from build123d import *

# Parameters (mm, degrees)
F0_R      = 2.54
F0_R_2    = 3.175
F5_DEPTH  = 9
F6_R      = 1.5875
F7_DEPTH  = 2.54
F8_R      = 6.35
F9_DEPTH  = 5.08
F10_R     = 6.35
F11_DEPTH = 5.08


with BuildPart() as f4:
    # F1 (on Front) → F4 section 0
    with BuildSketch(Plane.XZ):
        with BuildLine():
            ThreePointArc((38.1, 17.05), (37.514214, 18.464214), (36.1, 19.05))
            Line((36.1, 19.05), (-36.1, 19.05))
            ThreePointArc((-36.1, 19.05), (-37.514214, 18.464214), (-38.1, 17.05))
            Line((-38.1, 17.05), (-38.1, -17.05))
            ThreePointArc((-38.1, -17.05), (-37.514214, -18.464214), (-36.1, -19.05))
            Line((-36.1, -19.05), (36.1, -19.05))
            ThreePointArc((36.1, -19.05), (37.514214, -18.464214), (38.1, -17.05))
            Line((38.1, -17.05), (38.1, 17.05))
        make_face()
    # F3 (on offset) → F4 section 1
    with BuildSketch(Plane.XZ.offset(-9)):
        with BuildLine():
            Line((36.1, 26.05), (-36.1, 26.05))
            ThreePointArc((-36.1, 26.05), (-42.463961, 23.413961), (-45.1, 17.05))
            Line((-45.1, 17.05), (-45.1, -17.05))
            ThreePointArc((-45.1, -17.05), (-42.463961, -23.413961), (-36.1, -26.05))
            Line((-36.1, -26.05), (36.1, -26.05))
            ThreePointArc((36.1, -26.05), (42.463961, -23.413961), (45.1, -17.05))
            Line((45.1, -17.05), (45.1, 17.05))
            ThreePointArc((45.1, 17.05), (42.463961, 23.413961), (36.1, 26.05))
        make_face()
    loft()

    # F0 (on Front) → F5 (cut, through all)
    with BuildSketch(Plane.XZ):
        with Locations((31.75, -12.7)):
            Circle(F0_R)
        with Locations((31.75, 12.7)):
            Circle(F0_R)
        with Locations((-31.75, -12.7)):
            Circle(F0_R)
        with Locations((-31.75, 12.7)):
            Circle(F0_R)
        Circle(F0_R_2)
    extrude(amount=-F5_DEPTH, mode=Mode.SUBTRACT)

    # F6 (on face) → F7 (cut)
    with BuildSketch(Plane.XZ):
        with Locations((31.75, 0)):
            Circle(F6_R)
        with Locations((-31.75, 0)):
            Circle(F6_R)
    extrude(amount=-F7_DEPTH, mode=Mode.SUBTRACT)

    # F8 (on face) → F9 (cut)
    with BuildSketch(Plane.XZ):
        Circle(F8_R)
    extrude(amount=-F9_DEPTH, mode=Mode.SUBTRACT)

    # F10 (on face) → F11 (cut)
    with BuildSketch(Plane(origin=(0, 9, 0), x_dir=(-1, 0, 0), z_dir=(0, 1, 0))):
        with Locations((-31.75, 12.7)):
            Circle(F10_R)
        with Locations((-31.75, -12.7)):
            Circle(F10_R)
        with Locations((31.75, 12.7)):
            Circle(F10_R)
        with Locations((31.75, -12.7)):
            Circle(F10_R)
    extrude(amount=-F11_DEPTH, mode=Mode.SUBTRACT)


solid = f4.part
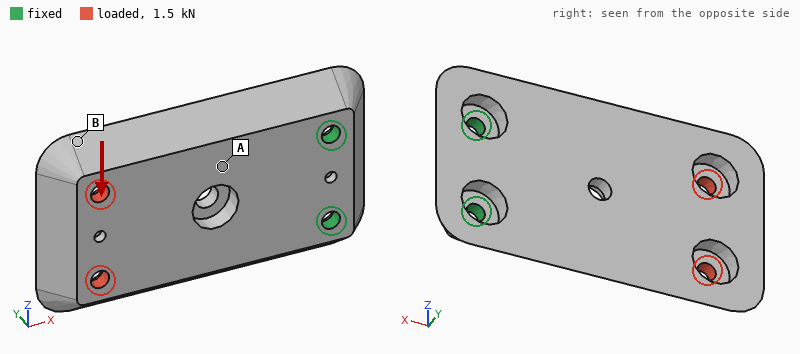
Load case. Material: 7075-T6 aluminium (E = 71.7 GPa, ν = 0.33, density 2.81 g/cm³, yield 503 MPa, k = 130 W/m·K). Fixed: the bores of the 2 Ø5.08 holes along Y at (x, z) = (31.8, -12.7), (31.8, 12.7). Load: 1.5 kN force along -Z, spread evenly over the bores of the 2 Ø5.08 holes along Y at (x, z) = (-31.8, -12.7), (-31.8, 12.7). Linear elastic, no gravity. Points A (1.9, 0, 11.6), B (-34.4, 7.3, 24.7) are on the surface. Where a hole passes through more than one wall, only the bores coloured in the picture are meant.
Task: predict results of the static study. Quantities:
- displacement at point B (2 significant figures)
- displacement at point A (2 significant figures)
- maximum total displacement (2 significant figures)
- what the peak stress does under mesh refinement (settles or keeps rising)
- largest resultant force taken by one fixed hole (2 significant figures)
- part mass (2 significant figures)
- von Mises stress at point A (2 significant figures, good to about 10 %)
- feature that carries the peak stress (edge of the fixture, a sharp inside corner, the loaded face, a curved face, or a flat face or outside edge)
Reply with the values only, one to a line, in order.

83 µm
35 µm
90 µm
keeps rising
3.4 kN
84 g
25 MPa
edge of the fixture
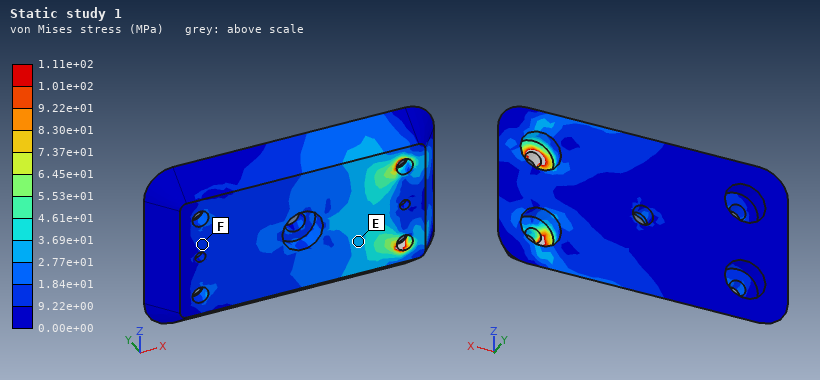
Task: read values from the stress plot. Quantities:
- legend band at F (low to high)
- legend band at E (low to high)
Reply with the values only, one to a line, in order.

9.22e+00 to 1.84e+01 MPa
2.77e+01 to 3.69e+01 MPa
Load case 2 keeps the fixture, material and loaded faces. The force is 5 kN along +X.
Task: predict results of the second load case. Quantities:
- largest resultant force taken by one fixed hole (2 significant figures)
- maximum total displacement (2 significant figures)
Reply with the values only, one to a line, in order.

2.5 kN
0.20 mm
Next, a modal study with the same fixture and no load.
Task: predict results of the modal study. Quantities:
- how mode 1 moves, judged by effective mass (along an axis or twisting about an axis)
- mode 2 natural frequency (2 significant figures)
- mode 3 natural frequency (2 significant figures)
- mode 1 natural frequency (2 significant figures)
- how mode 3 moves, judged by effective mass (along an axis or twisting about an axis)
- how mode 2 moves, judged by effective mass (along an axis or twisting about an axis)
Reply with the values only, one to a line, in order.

along Y
3800 Hz
4400 Hz
960 Hz
along Z
along Z
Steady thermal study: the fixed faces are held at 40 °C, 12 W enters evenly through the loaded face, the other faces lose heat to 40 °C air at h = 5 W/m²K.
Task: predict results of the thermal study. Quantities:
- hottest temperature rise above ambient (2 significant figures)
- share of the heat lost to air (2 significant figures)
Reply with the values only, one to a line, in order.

20 K
4.3 %
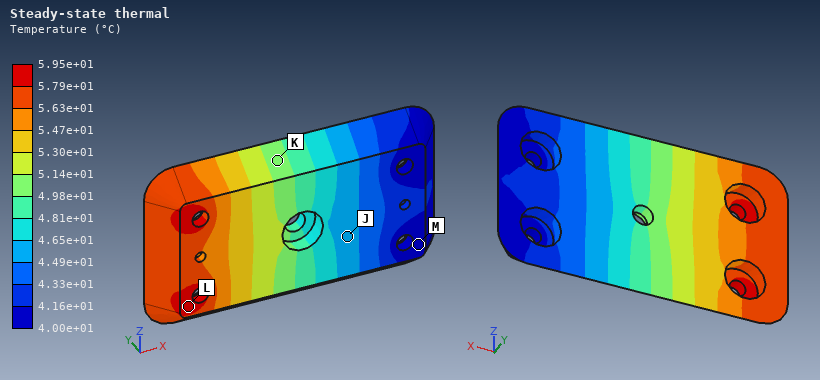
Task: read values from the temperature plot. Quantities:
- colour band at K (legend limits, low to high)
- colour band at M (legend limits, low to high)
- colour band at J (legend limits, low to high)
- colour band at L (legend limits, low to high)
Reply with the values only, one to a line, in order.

4.98e+01 to 5.14e+01 °C
4.00e+01 to 4.16e+01 °C
4.49e+01 to 4.65e+01 °C
5.79e+01 to 5.95e+01 °C
